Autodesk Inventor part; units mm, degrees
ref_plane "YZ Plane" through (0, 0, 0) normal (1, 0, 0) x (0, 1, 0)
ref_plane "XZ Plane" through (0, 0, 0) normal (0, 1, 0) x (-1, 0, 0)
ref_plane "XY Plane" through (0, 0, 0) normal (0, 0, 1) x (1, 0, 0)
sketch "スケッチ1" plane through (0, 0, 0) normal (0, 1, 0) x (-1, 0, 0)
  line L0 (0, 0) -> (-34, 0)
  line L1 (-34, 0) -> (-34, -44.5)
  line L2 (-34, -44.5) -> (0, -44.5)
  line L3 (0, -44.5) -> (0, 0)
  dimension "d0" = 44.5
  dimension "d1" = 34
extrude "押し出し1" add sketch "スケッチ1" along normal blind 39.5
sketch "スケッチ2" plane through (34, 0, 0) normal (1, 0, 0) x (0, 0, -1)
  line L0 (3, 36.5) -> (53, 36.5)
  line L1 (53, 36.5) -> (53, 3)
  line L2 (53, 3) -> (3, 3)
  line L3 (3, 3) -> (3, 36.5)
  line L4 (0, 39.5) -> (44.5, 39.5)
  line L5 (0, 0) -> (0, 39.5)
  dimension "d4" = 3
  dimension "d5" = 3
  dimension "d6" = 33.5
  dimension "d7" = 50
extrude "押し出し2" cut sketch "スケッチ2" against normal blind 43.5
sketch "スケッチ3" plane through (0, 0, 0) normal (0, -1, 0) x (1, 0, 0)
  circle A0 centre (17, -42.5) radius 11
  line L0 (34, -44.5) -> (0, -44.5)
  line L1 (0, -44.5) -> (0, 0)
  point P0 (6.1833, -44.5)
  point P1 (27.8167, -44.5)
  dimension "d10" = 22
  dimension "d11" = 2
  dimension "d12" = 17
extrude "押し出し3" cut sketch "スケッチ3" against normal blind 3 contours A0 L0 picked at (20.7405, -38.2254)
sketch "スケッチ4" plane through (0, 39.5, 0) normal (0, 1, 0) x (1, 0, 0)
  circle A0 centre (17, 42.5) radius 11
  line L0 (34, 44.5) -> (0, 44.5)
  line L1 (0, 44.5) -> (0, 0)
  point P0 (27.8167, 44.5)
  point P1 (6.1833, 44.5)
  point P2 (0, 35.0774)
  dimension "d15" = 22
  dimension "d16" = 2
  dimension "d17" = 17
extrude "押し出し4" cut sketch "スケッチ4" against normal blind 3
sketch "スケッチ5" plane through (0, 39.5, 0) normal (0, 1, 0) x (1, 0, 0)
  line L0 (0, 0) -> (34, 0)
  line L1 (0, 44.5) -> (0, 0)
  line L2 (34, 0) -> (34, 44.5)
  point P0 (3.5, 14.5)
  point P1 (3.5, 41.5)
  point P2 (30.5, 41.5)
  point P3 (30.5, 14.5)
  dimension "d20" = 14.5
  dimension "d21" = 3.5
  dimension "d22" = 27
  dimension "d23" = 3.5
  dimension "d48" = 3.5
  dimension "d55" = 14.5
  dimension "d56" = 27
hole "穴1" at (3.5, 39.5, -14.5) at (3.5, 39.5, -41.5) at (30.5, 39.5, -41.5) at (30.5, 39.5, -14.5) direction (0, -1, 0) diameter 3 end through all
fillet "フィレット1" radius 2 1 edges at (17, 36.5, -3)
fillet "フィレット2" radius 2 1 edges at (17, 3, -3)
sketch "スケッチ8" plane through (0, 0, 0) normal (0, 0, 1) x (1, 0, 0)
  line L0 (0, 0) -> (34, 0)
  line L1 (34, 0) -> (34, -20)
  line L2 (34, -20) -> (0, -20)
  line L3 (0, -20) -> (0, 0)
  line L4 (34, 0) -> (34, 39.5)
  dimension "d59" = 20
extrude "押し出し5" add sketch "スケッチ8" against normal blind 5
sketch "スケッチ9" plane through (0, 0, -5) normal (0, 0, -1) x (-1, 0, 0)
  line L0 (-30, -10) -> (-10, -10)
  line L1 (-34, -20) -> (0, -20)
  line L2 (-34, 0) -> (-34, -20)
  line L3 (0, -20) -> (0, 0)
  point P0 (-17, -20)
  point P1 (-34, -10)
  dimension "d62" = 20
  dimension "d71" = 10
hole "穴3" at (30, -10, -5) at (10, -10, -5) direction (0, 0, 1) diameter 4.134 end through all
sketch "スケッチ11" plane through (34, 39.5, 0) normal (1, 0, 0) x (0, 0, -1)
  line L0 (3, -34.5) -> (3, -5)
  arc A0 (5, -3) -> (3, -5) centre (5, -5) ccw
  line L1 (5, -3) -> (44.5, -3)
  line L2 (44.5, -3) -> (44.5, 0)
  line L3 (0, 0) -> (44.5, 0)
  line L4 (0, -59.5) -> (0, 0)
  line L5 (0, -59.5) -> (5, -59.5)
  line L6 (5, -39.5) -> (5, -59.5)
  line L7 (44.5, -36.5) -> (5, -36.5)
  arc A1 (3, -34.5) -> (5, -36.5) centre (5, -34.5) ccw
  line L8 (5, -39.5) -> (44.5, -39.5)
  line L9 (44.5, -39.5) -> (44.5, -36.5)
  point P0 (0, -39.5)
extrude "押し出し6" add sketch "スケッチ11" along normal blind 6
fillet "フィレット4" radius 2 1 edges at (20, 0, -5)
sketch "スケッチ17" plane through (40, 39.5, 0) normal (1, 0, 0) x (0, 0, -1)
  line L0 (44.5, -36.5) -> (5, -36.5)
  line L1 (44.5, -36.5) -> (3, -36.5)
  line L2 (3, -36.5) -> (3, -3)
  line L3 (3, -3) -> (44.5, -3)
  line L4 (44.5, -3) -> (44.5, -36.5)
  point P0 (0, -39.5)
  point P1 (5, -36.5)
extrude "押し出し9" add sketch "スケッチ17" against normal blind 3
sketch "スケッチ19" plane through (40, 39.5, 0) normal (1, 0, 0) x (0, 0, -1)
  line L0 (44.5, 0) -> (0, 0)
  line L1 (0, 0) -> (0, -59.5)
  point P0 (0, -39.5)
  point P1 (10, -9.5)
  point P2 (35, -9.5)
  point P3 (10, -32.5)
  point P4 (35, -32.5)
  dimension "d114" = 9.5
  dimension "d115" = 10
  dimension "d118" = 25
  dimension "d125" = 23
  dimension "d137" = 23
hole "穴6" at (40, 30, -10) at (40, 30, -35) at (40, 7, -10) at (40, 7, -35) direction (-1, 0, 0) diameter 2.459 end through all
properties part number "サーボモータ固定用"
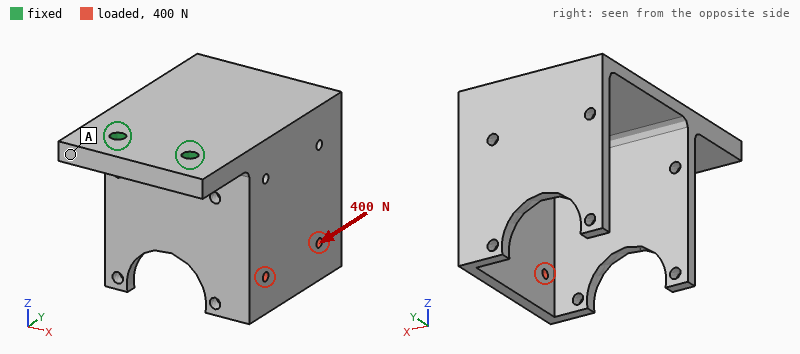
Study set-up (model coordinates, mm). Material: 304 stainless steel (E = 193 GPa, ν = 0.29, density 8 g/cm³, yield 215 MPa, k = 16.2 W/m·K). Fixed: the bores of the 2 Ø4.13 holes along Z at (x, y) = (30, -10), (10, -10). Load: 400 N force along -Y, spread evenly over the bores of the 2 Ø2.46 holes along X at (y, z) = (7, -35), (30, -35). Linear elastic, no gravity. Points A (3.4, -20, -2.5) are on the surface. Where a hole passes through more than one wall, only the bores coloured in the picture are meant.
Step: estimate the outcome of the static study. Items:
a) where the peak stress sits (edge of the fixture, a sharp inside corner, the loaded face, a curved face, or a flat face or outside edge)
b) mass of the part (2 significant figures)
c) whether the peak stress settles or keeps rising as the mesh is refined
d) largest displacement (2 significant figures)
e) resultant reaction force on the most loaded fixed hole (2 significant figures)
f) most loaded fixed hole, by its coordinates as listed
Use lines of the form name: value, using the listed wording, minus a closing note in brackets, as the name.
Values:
where the peak stress sits: edge of the fixture
mass of the part: 170 g
whether the peak stress settles or keeps rising as the mesh is refined: keeps rising
largest displacement: 0.22 mm
resultant reaction force on the most loaded fixed hole: 530 N
most loaded fixed hole, by its coordinates as listed: (30, -10)
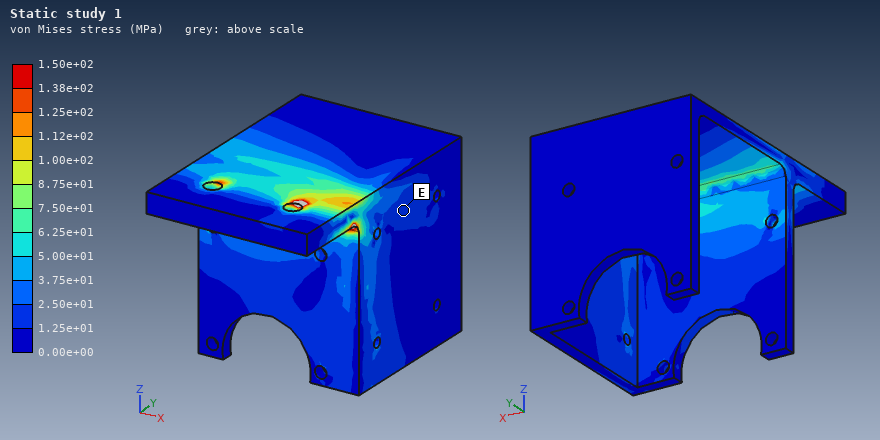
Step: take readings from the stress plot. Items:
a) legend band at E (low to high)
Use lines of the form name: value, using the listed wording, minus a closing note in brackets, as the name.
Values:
legend band at E: 1.25e+01 to 2.50e+01 MPa
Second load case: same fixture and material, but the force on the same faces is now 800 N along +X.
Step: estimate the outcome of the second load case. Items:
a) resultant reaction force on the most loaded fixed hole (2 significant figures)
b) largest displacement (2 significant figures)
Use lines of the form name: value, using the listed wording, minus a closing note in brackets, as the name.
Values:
resultant reaction force on the most loaded fixed hole: 1.5 kN
largest displacement: 0.23 mm
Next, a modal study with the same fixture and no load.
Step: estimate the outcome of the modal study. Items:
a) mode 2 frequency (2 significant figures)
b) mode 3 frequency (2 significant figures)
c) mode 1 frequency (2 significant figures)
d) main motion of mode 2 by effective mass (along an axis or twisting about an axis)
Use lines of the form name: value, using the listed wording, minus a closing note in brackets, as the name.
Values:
mode 2 frequency: 1400 Hz
mode 3 frequency: 2500 Hz
mode 1 frequency: 800 Hz
main motion of mode 2 by effective mass: along X
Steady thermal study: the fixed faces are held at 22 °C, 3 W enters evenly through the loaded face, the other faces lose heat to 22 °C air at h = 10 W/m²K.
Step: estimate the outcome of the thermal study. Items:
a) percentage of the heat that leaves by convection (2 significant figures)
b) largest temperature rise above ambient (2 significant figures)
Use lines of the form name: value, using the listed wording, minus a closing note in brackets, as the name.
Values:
percentage of the heat that leaves by convection: 58 %
largest temperature rise above ambient: 37 K
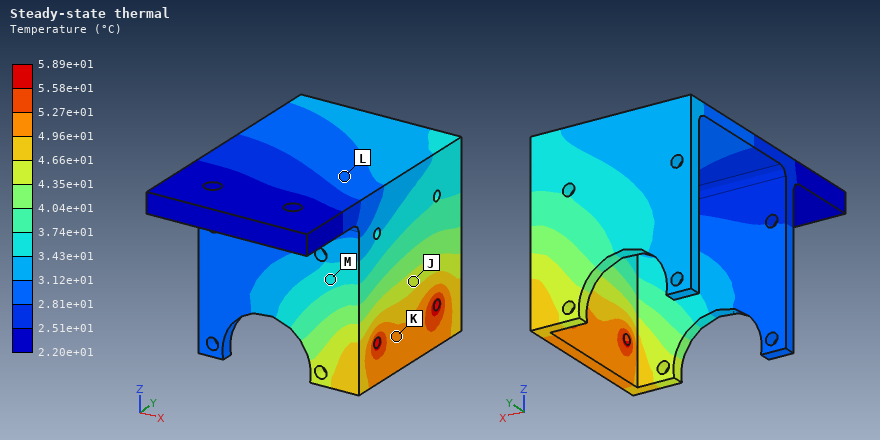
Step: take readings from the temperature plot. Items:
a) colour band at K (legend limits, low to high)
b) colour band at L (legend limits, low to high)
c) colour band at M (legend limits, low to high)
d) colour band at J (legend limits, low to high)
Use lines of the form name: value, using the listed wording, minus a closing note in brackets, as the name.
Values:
colour band at K: 4.96e+01 to 5.27e+01 °C
colour band at L: 2.81e+01 to 3.12e+01 °C
colour band at M: 3.43e+01 to 3.74e+01 °C
colour band at J: 4.35e+01 to 4.66e+01 °C
